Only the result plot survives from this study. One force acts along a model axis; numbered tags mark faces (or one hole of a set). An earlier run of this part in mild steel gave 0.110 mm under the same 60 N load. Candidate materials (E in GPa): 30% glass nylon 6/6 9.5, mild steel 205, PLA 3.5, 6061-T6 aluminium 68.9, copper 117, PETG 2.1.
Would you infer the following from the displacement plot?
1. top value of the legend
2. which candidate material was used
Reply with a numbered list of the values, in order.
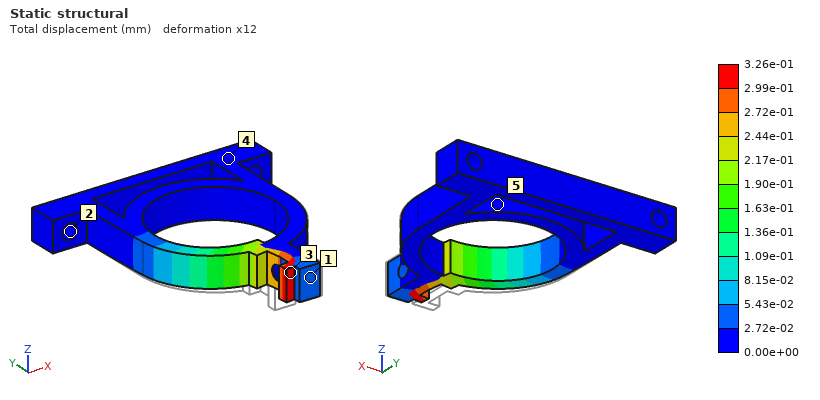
1. 3.26e-01 mm
2. 6061-T6 aluminium
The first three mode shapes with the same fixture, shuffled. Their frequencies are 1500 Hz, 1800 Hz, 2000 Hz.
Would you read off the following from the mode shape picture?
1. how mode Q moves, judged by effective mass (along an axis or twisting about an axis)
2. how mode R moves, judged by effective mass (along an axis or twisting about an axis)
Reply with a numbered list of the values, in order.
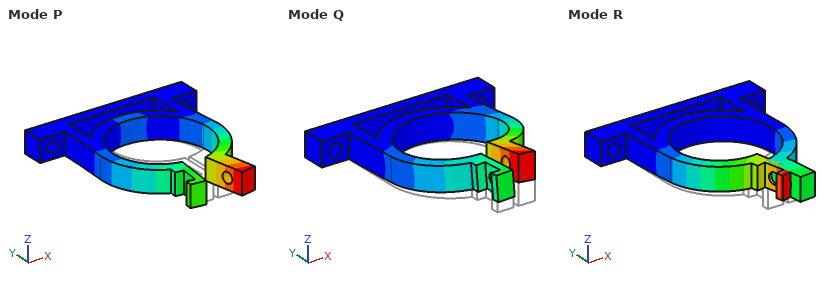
1. along Z
2. along X
